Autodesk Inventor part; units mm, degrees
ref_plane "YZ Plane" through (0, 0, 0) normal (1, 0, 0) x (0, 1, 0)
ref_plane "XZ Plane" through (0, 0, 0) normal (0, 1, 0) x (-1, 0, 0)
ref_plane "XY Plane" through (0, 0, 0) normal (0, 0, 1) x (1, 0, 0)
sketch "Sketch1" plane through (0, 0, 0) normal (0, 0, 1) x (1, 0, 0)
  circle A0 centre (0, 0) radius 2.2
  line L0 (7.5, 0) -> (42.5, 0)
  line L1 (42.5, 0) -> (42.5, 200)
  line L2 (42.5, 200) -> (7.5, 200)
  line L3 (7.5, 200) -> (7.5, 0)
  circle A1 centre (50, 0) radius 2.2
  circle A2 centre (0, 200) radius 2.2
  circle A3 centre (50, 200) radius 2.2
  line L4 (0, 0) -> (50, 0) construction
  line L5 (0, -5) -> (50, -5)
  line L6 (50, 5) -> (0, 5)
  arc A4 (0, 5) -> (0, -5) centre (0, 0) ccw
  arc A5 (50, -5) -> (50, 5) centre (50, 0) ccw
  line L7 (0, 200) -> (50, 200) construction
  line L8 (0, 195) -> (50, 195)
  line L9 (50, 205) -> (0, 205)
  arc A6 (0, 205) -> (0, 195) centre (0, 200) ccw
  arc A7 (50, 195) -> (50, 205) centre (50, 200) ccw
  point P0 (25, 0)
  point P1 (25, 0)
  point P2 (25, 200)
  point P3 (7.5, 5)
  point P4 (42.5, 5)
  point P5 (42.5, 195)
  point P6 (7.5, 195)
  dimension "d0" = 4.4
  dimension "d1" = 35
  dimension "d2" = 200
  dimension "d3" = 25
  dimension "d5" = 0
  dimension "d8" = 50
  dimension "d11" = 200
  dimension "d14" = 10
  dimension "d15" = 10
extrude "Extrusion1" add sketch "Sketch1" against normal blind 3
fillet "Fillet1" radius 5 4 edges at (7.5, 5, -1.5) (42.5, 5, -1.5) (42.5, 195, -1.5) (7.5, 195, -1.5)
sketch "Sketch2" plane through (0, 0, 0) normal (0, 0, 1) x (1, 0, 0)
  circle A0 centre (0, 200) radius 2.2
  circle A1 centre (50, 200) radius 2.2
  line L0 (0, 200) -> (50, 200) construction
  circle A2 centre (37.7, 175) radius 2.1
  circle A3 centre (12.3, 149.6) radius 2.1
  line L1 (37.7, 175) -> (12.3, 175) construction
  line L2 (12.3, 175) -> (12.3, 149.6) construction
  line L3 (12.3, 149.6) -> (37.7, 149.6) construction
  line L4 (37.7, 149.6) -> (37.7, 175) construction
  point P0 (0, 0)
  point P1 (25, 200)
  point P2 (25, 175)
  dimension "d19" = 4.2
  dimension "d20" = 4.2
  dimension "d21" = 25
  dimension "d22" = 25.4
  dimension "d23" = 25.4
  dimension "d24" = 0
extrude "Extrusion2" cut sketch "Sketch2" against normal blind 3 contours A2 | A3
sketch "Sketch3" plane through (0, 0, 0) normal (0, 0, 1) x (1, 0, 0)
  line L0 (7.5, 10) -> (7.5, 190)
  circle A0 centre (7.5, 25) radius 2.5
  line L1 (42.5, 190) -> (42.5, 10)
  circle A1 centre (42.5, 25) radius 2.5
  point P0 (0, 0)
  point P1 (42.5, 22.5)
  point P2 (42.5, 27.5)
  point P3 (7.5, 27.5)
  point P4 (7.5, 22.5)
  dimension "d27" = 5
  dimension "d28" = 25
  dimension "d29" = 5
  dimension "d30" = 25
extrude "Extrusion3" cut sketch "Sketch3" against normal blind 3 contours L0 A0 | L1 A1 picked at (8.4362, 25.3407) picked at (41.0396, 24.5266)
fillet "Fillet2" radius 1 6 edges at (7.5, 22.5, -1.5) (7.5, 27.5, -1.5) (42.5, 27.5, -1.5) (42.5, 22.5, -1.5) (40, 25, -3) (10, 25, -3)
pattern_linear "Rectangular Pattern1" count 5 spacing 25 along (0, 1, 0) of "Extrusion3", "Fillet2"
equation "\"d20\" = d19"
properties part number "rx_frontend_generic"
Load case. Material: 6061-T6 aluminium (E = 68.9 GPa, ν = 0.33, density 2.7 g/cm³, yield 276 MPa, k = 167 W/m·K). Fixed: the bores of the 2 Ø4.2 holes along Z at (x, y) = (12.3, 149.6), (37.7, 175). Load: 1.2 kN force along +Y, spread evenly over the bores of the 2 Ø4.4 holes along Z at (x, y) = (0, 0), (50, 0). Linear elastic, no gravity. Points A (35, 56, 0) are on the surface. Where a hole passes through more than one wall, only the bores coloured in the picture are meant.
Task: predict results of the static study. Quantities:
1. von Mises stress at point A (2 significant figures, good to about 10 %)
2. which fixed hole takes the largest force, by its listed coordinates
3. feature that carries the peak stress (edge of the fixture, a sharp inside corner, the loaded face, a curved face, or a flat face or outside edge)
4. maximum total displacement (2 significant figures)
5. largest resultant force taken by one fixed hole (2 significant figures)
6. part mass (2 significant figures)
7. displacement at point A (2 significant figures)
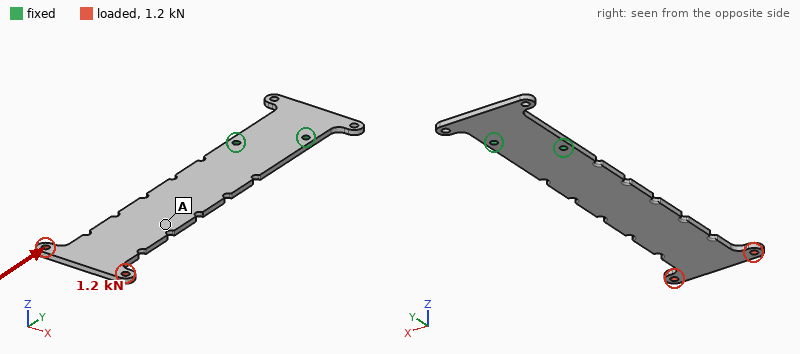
13 MPa
(12.3, 149.6)
a curved face
86 µm
670 N
62 g
29 µm
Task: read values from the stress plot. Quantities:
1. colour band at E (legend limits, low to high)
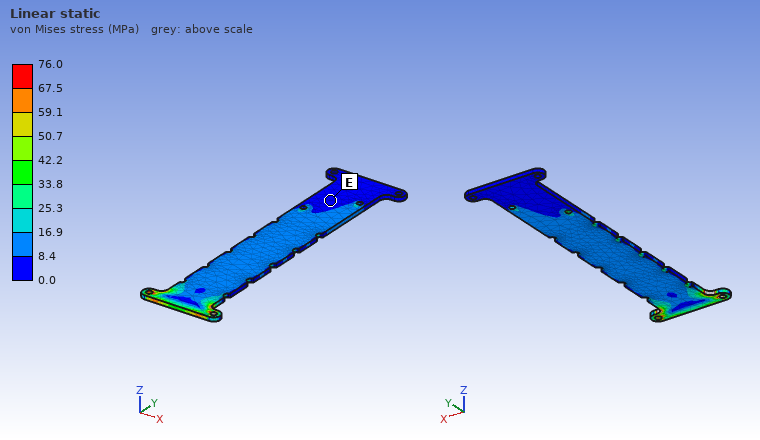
0.0 to 8.4 MPa
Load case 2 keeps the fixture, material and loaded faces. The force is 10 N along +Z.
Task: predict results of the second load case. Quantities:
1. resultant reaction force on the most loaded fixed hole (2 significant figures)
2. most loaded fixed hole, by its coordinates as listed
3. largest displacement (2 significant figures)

34 N
(12.3, 149.6)
2.4 mm
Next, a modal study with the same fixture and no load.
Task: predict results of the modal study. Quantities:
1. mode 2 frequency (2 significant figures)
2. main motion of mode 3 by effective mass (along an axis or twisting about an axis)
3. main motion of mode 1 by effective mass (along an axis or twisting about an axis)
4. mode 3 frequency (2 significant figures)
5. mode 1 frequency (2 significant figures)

570 Hz
twisting about Y
along Z
700 Hz
92 Hz
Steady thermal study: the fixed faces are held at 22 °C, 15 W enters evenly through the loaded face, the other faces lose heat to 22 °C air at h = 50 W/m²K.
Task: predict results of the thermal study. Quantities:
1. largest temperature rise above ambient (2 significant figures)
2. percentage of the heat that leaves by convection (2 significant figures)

65 K
85 %
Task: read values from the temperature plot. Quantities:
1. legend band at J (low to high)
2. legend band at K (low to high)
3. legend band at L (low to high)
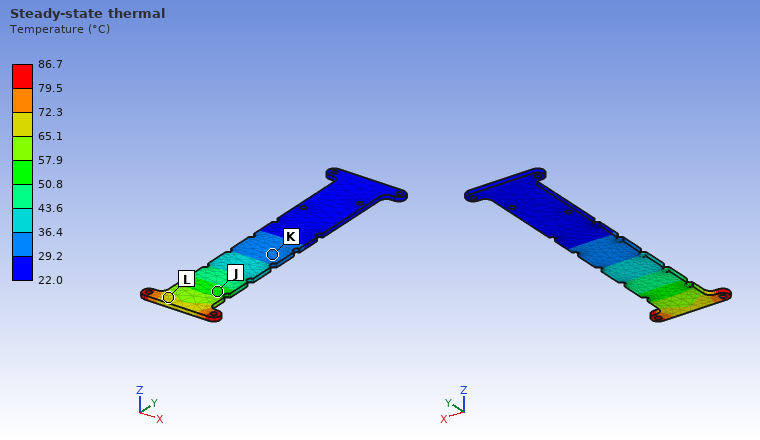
50.8 to 57.9 °C
29.2 to 36.4 °C
65.1 to 72.3 °C
